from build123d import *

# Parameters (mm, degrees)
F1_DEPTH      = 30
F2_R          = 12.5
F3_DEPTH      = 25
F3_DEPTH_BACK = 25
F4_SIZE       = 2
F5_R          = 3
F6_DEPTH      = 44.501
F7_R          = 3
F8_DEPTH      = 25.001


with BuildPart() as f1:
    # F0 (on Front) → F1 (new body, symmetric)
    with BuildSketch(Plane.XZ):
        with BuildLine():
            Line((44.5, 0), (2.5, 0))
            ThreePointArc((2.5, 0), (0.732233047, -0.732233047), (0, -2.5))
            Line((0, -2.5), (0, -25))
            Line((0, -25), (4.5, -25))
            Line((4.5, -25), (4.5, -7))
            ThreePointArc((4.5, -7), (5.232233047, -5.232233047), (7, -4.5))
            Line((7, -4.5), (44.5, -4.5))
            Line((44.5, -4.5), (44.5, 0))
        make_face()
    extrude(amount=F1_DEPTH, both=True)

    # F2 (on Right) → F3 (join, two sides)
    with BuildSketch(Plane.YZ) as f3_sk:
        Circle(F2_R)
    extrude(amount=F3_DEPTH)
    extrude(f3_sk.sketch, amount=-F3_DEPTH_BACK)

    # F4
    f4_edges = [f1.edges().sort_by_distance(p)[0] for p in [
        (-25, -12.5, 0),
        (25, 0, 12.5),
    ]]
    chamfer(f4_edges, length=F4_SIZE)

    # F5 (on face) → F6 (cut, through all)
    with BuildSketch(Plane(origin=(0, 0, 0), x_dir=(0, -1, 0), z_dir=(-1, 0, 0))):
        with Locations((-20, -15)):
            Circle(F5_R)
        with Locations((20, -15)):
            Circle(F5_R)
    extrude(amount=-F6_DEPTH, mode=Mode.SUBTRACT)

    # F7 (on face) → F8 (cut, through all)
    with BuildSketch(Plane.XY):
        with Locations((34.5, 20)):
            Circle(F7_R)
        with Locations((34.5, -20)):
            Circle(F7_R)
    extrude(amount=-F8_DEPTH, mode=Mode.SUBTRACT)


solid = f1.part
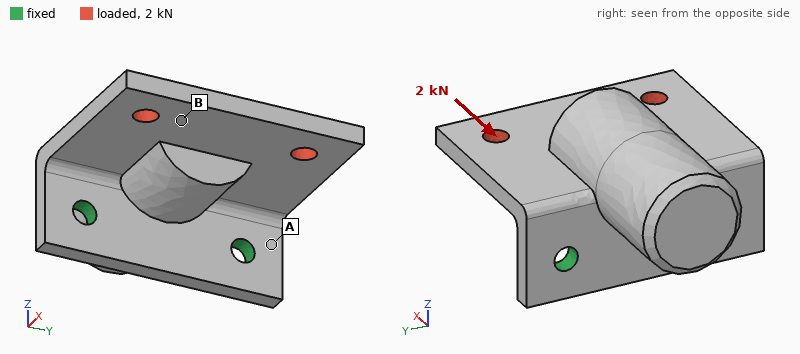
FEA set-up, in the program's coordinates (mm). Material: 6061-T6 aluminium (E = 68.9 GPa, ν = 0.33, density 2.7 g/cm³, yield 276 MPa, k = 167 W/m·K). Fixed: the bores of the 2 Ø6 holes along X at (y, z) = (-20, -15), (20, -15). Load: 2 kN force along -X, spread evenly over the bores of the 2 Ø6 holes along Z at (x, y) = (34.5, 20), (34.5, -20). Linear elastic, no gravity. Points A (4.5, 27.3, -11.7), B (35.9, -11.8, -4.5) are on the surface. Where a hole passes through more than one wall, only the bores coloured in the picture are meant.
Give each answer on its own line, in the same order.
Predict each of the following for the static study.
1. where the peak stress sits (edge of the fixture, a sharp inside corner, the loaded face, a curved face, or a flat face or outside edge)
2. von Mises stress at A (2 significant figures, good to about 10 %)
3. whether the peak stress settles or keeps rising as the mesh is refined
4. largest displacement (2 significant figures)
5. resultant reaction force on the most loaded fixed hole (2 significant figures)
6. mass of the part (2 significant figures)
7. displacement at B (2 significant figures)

edge of the fixture
61 MPa
keeps rising
0.18 mm
1.0 kN
100 g
0.14 mm
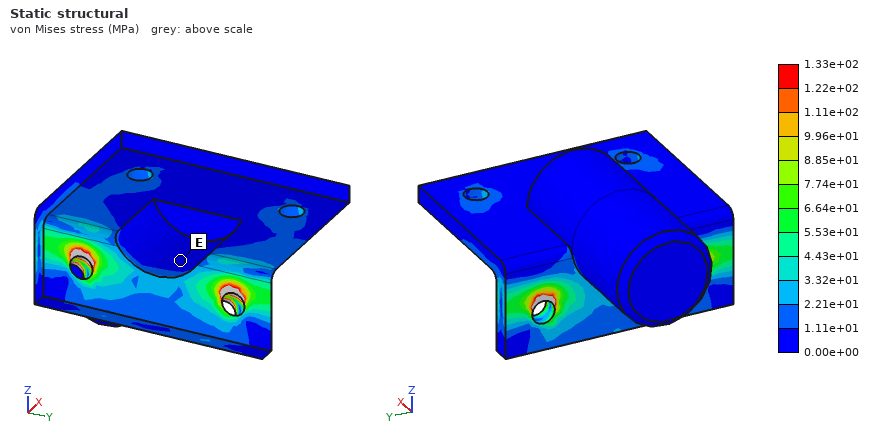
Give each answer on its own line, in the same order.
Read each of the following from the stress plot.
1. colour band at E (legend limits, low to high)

0.00e+00 to 1.11e+01 MPa
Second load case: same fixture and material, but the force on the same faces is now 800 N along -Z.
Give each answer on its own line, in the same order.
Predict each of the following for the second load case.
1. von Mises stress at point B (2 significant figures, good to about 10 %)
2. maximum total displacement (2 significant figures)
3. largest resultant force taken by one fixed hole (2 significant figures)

17 MPa
0.37 mm
420 N
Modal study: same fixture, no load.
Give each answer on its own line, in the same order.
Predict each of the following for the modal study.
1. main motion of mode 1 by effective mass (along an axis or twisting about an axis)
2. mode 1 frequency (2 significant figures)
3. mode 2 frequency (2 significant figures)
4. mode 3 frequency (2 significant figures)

along X
1500 Hz
4800 Hz
6100 Hz
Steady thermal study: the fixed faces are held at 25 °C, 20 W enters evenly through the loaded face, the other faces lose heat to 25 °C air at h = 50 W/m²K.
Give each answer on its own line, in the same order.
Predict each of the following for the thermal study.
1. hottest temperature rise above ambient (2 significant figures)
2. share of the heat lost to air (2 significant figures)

17 K
20 %
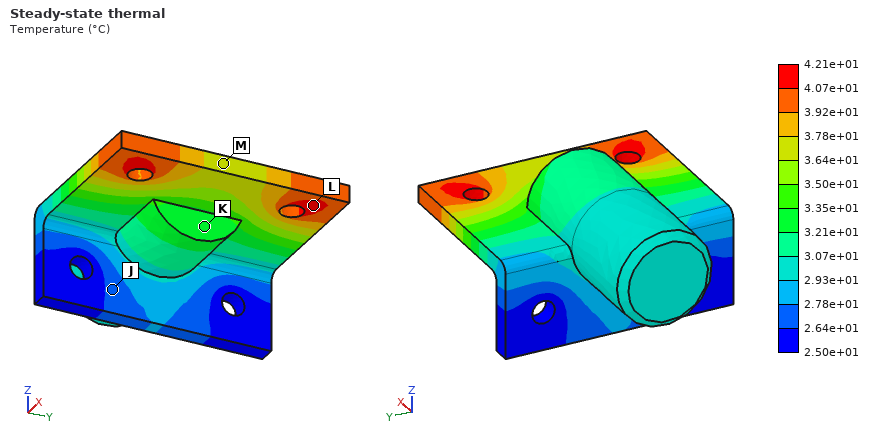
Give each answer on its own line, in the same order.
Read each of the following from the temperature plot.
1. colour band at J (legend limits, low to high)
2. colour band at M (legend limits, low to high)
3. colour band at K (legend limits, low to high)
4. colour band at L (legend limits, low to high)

2.64e+01 to 2.78e+01 °C
3.64e+01 to 3.78e+01 °C
3.21e+01 to 3.35e+01 °C
4.07e+01 to 4.21e+01 °C
